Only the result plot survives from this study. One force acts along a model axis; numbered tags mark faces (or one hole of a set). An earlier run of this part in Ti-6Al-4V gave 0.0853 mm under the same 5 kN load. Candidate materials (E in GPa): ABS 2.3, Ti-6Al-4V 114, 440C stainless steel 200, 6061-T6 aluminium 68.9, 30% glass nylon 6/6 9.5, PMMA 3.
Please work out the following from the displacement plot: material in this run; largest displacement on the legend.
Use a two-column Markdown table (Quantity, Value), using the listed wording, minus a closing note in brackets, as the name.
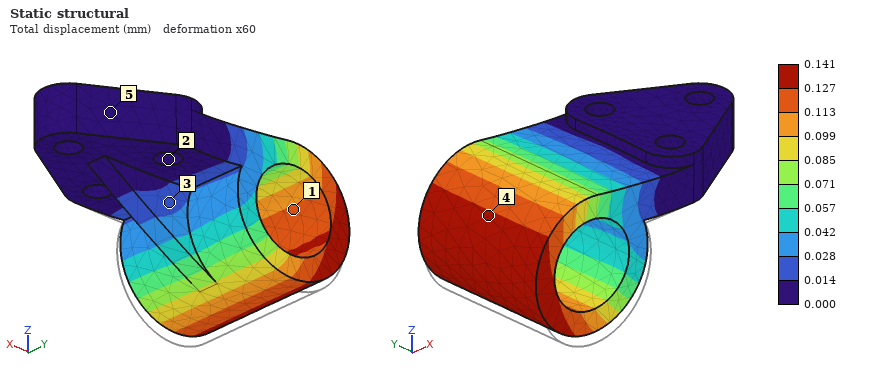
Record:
| Quantity | Value |
|---|---|
| material in this run | 6061-T6 aluminium |
| largest displacement on the legend | 0.141 mm |
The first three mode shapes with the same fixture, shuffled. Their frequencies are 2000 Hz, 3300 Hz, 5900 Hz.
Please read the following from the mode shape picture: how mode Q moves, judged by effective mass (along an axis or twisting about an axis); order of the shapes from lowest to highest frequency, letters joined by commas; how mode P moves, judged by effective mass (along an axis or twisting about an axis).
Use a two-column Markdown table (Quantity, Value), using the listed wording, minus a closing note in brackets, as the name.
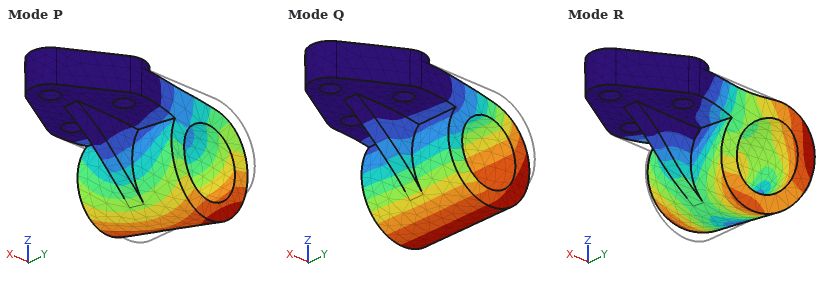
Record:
| Quantity | Value |
|---|---|
| how mode Q moves, judged by effective mass | along Z |
| order of the shapes from lowest to highest frequency, letters joined by commas | Q, P, R |
| how mode P moves, judged by effective mass | along Y |
